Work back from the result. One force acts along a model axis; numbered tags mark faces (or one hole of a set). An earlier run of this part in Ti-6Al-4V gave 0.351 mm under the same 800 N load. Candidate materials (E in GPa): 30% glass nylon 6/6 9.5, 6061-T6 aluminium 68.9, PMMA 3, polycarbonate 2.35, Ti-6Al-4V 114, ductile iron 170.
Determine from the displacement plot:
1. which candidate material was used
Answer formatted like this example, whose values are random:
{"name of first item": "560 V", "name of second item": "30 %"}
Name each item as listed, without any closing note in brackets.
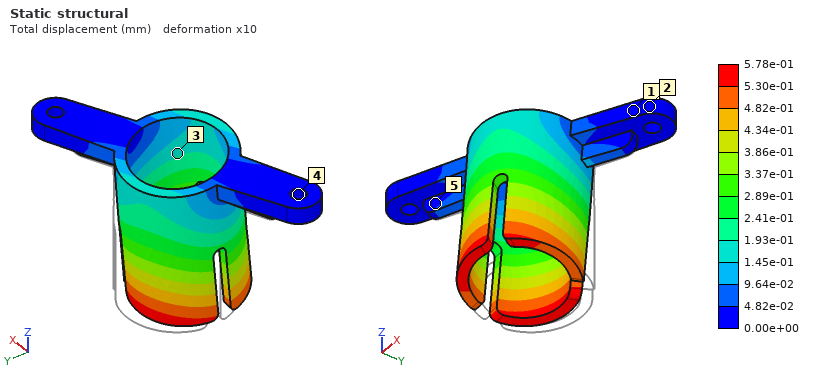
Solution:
{"which candidate material was used": "6061-T6 aluminium"}
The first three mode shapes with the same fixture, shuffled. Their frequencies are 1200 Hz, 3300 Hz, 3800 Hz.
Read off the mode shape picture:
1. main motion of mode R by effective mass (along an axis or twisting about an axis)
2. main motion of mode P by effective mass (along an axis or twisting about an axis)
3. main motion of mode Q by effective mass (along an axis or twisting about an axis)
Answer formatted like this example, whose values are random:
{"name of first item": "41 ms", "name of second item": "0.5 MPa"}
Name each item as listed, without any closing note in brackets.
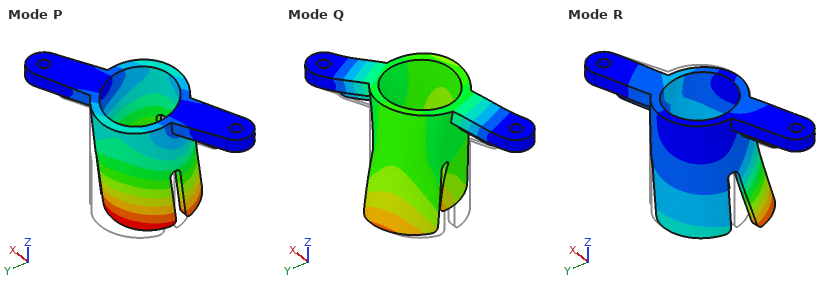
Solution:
{"main motion of mode R by effective mass": "along X", "main motion of mode P by effective mass": "along Y", "main motion of mode Q by effective mass": "along Z"}
